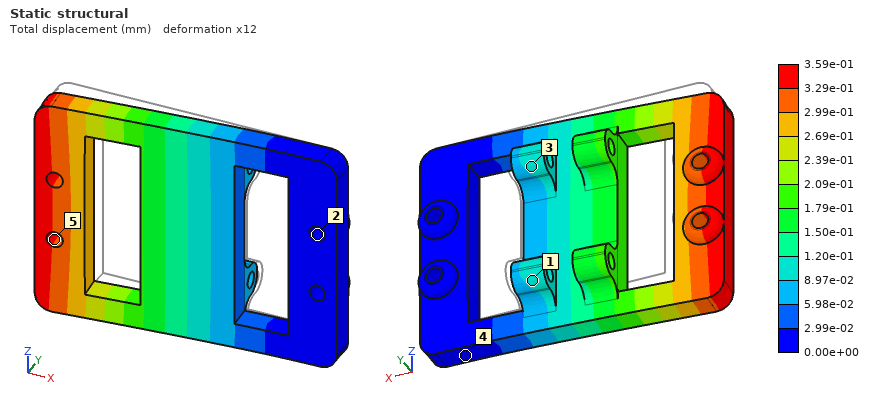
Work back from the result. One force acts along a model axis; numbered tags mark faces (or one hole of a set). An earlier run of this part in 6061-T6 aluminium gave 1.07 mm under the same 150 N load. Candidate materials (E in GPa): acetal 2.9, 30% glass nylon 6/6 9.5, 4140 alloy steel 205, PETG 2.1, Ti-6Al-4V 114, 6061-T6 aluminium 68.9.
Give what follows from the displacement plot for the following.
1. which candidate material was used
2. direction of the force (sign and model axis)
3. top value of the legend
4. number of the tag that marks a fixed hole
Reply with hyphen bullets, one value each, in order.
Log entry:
- 4140 alloy steel
- -Y
- 3.59e-01 mm
- 2
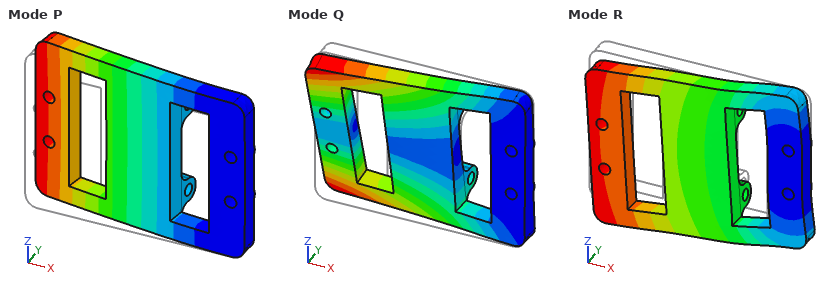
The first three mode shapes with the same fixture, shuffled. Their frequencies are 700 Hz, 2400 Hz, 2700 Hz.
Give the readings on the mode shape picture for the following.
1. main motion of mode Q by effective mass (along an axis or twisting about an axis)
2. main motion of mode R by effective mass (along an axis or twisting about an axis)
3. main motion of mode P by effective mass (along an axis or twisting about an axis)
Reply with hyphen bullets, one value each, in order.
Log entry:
- twisting about X
- along Z
- along Y
